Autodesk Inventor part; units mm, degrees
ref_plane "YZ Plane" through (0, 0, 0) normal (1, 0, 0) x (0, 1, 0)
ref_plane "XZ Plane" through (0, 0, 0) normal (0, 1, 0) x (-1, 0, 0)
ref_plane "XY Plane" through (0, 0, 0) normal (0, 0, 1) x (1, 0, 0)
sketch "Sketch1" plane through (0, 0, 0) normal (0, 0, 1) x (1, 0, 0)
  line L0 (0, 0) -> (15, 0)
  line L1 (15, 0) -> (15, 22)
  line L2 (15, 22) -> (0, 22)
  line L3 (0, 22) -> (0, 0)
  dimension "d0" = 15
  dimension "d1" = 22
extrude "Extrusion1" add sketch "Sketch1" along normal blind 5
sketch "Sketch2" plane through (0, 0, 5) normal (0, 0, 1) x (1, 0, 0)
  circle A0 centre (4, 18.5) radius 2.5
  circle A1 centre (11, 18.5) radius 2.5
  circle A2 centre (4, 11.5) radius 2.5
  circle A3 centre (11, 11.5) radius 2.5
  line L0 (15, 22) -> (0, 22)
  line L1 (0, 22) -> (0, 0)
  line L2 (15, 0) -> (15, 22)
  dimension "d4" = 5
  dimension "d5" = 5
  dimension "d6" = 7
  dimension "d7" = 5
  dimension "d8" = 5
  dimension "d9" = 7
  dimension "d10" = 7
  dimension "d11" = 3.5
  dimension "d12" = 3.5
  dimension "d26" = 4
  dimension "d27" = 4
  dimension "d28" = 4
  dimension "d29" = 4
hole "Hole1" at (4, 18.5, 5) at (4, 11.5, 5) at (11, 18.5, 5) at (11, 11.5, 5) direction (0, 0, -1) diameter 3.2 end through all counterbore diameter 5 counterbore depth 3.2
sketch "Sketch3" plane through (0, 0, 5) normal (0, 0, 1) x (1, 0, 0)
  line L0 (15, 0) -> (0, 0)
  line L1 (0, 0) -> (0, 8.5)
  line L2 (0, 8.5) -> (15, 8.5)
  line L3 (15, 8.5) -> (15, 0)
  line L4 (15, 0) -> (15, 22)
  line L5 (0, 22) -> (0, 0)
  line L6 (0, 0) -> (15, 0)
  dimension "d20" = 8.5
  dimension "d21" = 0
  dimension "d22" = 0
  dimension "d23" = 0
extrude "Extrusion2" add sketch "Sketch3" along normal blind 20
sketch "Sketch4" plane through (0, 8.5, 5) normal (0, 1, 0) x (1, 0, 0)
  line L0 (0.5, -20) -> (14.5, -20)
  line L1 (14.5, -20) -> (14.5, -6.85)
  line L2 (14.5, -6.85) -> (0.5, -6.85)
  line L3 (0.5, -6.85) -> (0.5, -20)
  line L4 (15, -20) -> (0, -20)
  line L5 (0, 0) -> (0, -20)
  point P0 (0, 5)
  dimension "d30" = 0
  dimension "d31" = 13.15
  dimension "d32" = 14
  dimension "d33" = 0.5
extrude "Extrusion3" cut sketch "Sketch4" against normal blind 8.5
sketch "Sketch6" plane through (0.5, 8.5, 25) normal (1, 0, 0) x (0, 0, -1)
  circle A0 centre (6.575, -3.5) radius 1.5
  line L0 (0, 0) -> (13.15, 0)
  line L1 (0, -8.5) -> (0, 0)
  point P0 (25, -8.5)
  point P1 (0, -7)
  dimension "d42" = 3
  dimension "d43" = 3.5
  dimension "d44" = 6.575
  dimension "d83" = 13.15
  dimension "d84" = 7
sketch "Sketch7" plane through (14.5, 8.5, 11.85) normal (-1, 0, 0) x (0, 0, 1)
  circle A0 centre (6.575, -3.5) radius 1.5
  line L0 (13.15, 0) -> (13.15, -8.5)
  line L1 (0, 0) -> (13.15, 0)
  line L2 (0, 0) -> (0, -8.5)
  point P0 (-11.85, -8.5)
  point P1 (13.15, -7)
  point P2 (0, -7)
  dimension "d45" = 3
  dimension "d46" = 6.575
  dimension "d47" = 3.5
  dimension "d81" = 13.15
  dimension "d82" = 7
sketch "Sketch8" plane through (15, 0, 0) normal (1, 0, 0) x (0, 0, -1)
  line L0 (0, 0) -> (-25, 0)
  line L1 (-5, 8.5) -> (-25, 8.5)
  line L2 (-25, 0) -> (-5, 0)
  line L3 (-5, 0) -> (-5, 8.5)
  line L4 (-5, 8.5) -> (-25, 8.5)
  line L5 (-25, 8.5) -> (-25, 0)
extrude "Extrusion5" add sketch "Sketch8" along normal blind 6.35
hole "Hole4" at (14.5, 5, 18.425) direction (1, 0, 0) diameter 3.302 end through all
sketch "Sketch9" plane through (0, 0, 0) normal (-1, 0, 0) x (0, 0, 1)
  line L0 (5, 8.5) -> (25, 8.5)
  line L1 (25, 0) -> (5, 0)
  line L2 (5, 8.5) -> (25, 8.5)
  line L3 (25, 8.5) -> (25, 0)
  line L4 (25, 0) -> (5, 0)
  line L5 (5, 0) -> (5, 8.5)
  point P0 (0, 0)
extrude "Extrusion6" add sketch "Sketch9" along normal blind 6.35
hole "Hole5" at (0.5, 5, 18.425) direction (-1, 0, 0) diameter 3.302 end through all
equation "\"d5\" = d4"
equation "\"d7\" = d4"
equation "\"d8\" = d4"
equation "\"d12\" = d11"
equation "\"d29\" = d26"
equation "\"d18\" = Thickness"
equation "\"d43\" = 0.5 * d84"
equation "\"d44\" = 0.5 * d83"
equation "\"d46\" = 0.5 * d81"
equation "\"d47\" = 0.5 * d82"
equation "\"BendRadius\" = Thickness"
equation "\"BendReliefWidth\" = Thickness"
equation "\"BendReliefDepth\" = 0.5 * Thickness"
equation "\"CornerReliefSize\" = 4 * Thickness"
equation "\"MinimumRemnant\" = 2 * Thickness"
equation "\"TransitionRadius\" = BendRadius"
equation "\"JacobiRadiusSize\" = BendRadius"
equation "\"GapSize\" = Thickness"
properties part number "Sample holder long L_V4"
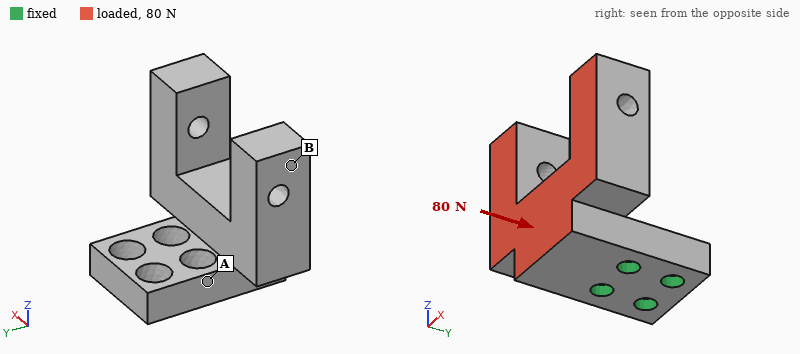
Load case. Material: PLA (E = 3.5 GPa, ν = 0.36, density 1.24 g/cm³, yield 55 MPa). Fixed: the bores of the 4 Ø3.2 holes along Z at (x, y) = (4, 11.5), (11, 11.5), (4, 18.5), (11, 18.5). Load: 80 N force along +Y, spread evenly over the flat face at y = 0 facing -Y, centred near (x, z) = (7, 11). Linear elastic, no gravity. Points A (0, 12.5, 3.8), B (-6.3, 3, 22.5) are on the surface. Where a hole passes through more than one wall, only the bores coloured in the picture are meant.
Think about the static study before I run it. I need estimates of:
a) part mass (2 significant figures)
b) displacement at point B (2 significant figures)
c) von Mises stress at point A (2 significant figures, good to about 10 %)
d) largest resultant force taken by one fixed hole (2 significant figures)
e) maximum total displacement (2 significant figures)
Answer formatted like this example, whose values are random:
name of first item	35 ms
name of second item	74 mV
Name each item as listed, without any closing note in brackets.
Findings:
part mass	5.4 g
displacement at point B	0.33 mm
von Mises stress at point A	9.2 MPa
largest resultant force taken by one fixed hole	63 N
maximum total displacement	0.38 mm
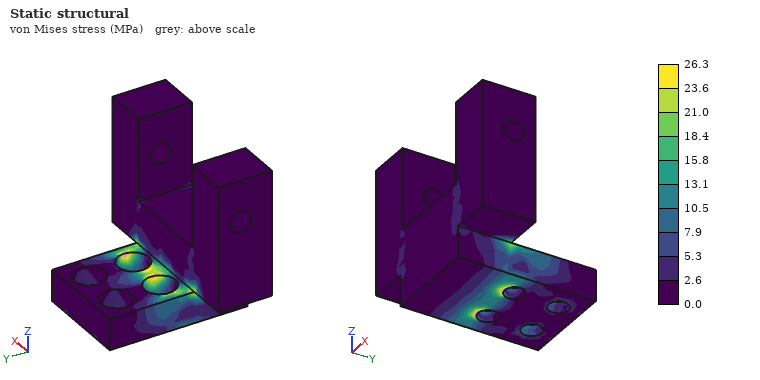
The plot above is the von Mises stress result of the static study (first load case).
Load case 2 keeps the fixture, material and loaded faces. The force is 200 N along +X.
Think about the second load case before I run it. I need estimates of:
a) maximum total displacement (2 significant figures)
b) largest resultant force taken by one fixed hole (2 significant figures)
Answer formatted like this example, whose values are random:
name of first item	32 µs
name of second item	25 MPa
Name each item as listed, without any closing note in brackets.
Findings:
maximum total displacement	0.42 mm
largest resultant force taken by one fixed hole	310 N
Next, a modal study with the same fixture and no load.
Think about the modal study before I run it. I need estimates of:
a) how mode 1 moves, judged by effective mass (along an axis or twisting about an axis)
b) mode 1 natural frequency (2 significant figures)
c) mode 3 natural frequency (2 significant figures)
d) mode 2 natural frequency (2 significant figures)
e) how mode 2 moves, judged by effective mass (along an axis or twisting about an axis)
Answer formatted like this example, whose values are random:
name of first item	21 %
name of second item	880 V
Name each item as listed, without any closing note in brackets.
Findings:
how mode 1 moves, judged by effective mass	along Y
mode 1 natural frequency	1300 Hz
mode 3 natural frequency	3100 Hz
mode 2 natural frequency	1900 Hz
how mode 2 moves, judged by effective mass	along X
